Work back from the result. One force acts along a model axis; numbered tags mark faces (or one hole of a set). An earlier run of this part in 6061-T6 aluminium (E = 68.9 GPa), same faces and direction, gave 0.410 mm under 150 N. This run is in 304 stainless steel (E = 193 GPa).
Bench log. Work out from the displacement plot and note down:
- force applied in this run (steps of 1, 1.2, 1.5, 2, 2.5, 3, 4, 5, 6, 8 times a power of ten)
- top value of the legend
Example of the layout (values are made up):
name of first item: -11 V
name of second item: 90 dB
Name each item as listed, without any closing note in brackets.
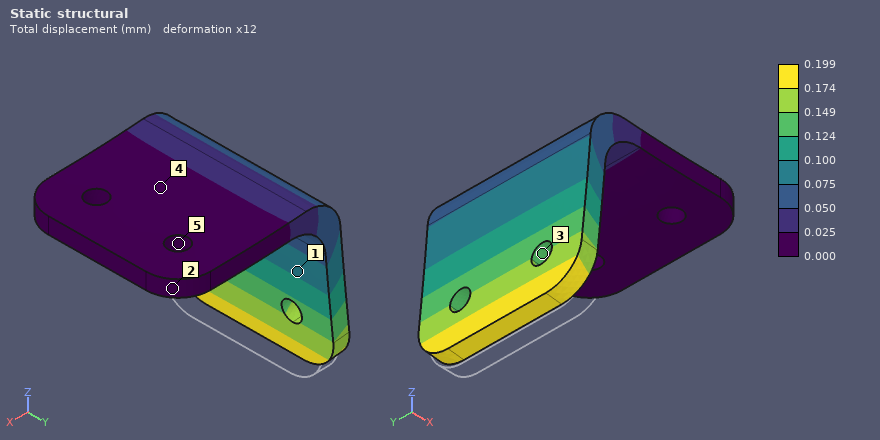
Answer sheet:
force applied in this run: 200 N
top value of the legend: 0.199 mm
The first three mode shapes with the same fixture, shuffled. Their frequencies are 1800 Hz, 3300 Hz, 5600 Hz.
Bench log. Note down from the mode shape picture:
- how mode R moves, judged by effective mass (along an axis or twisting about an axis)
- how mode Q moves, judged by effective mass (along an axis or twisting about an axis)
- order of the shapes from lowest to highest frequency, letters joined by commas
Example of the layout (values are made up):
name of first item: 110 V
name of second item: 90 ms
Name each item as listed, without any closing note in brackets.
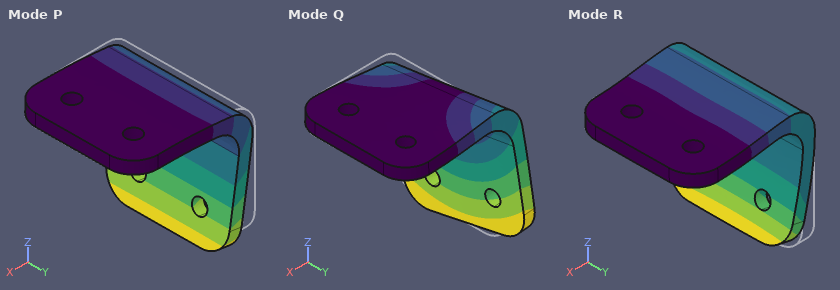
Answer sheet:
how mode R moves, judged by effective mass: along Z
how mode Q moves, judged by effective mass: along Y
order of the shapes from lowest to highest frequency, letters joined by commas: P, Q, R
